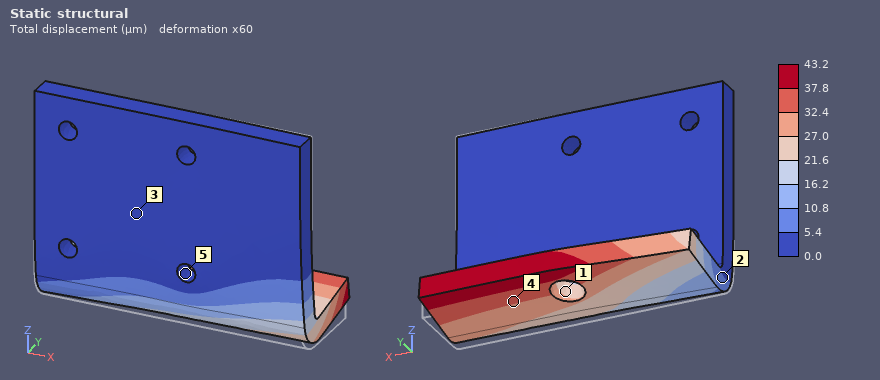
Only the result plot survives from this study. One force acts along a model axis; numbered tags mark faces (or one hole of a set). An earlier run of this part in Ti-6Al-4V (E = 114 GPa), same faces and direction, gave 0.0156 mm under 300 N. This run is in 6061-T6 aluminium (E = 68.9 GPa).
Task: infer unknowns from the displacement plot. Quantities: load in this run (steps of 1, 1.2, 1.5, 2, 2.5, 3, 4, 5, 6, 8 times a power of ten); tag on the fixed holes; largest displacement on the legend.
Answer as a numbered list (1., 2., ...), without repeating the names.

1. 500 N
2. 5
3. 43.2 µm
